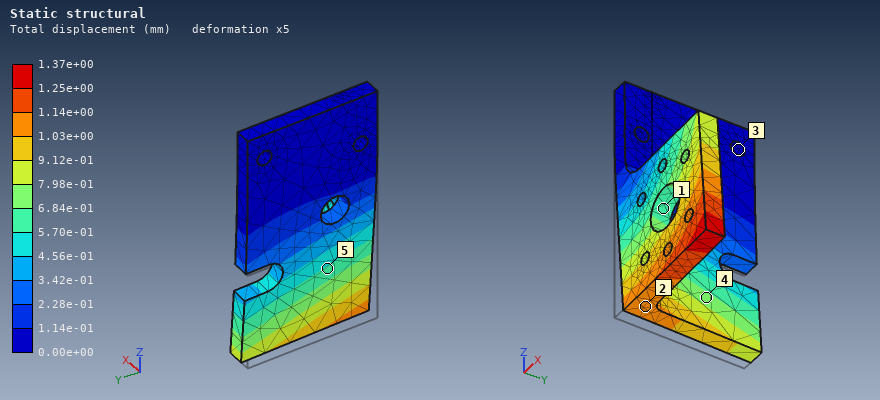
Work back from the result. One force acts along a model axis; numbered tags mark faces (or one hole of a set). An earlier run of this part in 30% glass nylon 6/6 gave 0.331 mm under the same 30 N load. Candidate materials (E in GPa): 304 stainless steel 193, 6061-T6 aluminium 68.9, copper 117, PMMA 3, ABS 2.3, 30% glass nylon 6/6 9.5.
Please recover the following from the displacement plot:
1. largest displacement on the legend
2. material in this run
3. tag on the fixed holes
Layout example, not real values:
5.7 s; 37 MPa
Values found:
1.37e+00 mm; ABS; 3
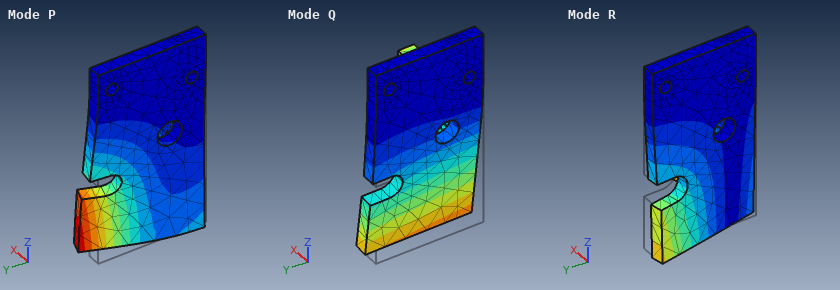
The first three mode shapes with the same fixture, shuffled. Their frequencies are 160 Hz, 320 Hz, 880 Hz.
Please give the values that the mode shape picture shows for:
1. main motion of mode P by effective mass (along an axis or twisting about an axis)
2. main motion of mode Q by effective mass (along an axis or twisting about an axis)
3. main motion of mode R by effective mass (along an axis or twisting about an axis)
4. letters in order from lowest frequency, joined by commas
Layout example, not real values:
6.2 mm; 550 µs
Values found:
along Y; along X; along Y; Q, R, P
